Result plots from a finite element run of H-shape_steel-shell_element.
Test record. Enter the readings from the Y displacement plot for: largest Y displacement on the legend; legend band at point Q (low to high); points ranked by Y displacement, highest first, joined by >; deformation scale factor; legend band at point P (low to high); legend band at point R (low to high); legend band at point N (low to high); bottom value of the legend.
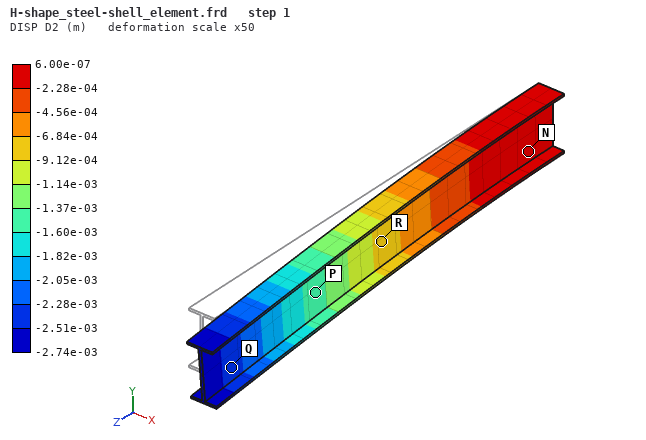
6.00e-07 m
-2.51e-03 to -2.28e-03 m
N > R > P > Q
50
-1.60e-03 to -1.37e-03 m
-9.12e-04 to -6.84e-04 m
-2.28e-04 to 6.00e-07 m
-2.74e-03 m
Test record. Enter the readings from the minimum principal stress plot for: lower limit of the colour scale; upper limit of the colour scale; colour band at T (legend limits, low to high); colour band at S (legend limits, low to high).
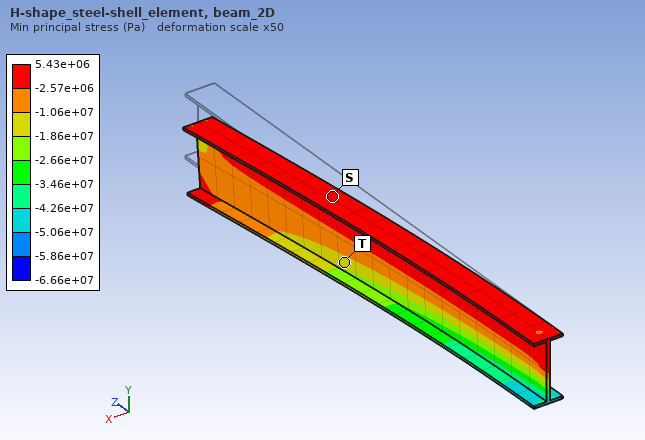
-6.66e+07 Pa
5.43e+06 Pa
-1.86e+07 to -1.06e+07 Pa
-2.57e+06 to 5.43e+06 Pa
